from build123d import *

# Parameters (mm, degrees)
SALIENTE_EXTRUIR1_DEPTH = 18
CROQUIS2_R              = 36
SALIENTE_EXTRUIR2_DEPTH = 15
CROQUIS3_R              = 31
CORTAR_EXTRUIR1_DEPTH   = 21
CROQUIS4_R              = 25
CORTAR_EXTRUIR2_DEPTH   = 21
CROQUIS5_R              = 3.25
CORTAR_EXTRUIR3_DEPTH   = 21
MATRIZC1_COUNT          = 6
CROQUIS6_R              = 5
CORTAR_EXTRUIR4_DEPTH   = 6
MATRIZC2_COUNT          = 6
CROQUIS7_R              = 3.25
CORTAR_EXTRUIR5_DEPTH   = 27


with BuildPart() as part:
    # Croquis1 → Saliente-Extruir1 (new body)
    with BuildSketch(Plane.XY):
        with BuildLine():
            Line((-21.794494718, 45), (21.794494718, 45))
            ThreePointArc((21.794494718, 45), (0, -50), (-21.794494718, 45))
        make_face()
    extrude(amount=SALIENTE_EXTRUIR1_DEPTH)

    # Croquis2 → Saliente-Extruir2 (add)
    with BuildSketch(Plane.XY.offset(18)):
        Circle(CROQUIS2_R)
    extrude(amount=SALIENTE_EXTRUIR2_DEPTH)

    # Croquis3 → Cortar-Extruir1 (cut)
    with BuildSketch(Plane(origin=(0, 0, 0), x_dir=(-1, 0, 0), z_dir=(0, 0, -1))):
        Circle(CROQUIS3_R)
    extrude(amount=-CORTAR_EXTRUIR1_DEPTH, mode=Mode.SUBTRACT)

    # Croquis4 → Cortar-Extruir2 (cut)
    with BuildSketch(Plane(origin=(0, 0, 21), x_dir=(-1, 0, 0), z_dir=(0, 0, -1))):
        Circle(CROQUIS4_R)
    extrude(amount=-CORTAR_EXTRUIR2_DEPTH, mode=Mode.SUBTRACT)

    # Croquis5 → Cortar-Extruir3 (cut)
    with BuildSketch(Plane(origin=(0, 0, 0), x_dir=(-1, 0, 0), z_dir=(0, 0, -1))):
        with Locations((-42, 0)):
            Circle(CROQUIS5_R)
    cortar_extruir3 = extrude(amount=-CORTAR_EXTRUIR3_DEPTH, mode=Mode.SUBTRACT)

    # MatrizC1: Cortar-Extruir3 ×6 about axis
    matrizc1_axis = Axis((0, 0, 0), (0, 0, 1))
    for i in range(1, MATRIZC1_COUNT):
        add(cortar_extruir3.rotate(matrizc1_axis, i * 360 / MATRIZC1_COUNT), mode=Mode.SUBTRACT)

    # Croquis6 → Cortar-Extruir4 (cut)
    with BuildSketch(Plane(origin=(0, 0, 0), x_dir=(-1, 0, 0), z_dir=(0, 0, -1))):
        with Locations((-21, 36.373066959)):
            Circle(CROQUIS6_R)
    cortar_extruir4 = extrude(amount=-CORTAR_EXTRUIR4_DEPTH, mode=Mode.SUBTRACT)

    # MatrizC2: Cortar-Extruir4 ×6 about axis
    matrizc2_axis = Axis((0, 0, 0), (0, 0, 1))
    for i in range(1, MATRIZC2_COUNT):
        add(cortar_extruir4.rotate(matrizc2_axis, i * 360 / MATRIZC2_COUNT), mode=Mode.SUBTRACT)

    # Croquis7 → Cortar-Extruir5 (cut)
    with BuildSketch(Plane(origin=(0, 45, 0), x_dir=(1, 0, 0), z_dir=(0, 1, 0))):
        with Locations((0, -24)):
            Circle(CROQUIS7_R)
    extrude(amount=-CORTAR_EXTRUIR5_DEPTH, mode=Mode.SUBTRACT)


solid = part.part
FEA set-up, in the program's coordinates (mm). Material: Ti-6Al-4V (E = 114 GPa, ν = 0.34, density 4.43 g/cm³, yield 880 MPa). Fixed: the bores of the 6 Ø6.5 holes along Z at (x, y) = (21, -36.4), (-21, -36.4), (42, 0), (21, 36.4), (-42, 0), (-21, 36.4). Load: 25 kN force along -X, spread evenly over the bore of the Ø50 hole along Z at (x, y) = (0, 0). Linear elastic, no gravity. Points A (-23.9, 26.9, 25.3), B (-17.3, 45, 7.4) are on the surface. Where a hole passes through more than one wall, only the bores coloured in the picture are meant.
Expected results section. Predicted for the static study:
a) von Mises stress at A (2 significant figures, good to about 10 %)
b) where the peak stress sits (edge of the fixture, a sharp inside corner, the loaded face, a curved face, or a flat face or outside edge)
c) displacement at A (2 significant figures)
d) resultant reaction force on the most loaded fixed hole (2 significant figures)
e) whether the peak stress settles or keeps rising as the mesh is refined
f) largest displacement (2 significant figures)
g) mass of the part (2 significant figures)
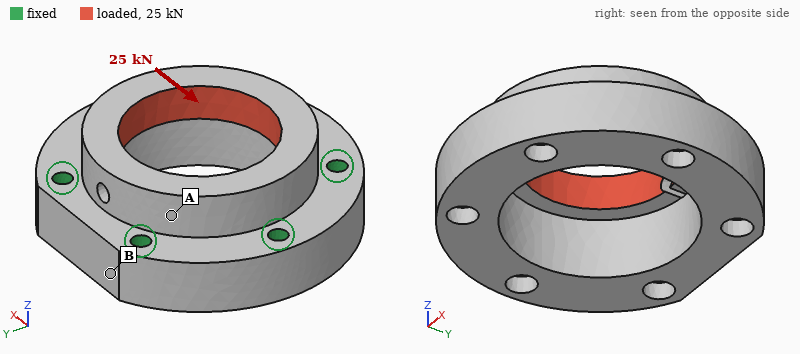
20 MPa
a sharp inside corner
11 µm
4.9 kN
keeps rising
26 µm
480 g
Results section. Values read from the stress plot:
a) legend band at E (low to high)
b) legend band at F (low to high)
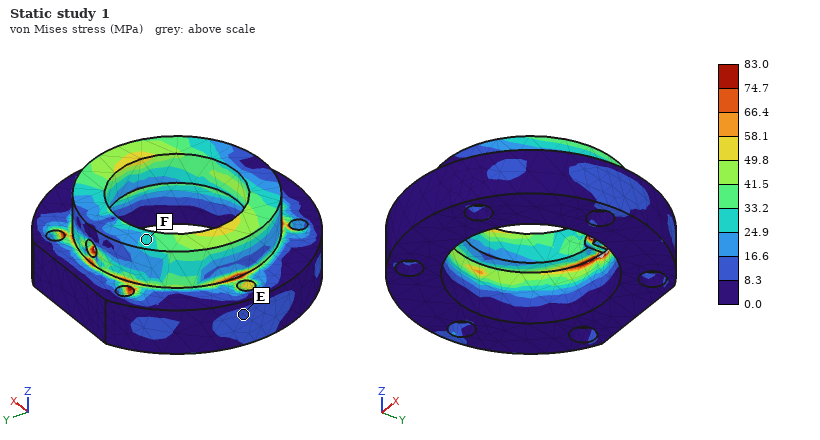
8.3 to 16.6 MPa
24.9 to 33.2 MPa
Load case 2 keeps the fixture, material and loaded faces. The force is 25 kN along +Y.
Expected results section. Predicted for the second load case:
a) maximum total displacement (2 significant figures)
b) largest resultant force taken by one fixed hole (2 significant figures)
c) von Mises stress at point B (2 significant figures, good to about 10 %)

25 µm
4.7 kN
14 MPa
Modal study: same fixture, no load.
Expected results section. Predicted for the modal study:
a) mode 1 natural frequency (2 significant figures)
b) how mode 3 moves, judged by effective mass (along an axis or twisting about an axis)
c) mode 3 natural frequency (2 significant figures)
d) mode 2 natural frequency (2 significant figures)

18 kHz
along X
19 kHz
18 kHz
